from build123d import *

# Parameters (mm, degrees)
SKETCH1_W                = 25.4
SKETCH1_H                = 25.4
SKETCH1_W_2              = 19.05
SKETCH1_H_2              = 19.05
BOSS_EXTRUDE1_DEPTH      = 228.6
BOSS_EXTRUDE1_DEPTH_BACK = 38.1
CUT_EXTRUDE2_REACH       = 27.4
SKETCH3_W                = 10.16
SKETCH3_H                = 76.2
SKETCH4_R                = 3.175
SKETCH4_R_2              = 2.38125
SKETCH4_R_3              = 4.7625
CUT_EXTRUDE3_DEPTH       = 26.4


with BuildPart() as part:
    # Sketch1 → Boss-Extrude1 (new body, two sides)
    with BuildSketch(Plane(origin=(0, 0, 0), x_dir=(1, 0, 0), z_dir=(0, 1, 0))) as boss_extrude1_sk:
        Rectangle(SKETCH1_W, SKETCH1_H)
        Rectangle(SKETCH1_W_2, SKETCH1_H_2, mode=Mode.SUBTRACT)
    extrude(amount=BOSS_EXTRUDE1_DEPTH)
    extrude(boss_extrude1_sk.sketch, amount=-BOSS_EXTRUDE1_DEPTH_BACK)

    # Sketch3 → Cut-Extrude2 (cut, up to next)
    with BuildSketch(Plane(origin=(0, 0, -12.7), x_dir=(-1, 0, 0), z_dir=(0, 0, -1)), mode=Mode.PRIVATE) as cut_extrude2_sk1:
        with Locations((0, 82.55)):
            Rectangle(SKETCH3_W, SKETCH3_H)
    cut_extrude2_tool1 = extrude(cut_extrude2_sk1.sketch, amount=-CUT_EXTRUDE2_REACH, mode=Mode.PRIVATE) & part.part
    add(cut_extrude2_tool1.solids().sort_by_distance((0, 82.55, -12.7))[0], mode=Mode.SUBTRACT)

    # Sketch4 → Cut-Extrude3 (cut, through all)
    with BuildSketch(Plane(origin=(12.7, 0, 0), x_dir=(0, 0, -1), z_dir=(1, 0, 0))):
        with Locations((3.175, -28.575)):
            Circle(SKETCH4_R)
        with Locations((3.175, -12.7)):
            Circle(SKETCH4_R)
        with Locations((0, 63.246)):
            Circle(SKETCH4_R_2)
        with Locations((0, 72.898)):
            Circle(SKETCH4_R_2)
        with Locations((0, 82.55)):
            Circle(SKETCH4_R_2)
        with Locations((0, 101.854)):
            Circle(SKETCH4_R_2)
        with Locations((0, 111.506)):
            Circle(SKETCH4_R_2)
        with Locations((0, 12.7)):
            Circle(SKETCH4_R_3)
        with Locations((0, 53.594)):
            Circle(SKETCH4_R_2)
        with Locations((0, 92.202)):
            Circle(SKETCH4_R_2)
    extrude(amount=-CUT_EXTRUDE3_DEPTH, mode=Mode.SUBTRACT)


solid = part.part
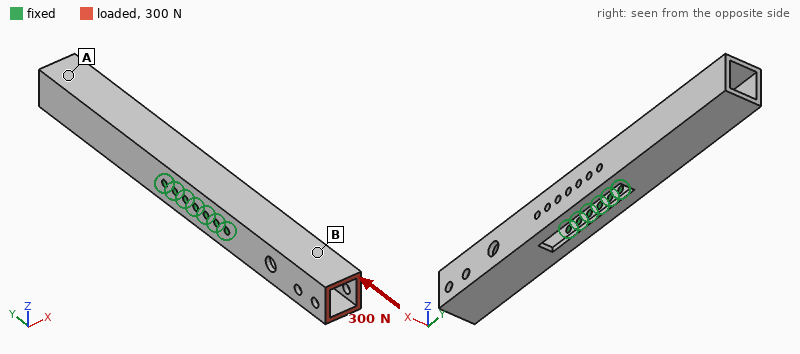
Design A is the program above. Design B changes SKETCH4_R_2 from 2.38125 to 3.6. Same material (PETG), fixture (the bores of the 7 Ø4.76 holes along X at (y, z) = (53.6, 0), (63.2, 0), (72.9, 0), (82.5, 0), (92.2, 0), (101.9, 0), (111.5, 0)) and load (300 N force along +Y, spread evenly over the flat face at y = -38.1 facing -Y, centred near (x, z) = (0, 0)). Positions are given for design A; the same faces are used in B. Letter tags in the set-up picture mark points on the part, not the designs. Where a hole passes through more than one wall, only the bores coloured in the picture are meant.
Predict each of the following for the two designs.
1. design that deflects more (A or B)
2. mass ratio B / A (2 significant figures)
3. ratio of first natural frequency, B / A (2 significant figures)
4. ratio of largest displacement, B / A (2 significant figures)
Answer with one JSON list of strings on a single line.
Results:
["A", "0.99", "1.1", "0.83"]
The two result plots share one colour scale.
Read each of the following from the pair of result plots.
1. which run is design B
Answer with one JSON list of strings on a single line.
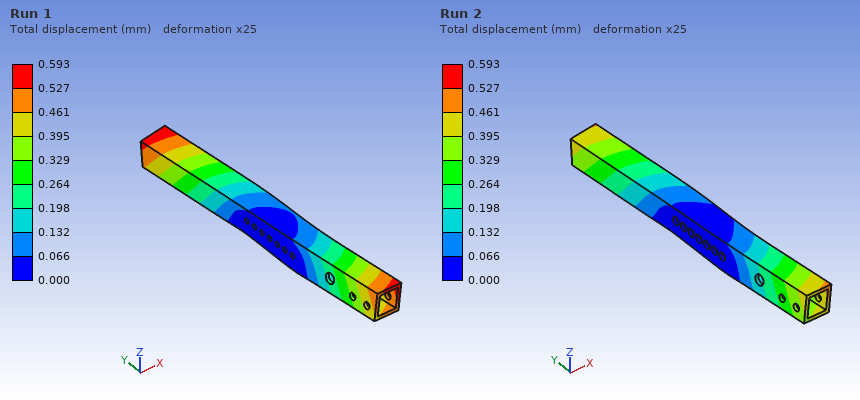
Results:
["Run 2"]
